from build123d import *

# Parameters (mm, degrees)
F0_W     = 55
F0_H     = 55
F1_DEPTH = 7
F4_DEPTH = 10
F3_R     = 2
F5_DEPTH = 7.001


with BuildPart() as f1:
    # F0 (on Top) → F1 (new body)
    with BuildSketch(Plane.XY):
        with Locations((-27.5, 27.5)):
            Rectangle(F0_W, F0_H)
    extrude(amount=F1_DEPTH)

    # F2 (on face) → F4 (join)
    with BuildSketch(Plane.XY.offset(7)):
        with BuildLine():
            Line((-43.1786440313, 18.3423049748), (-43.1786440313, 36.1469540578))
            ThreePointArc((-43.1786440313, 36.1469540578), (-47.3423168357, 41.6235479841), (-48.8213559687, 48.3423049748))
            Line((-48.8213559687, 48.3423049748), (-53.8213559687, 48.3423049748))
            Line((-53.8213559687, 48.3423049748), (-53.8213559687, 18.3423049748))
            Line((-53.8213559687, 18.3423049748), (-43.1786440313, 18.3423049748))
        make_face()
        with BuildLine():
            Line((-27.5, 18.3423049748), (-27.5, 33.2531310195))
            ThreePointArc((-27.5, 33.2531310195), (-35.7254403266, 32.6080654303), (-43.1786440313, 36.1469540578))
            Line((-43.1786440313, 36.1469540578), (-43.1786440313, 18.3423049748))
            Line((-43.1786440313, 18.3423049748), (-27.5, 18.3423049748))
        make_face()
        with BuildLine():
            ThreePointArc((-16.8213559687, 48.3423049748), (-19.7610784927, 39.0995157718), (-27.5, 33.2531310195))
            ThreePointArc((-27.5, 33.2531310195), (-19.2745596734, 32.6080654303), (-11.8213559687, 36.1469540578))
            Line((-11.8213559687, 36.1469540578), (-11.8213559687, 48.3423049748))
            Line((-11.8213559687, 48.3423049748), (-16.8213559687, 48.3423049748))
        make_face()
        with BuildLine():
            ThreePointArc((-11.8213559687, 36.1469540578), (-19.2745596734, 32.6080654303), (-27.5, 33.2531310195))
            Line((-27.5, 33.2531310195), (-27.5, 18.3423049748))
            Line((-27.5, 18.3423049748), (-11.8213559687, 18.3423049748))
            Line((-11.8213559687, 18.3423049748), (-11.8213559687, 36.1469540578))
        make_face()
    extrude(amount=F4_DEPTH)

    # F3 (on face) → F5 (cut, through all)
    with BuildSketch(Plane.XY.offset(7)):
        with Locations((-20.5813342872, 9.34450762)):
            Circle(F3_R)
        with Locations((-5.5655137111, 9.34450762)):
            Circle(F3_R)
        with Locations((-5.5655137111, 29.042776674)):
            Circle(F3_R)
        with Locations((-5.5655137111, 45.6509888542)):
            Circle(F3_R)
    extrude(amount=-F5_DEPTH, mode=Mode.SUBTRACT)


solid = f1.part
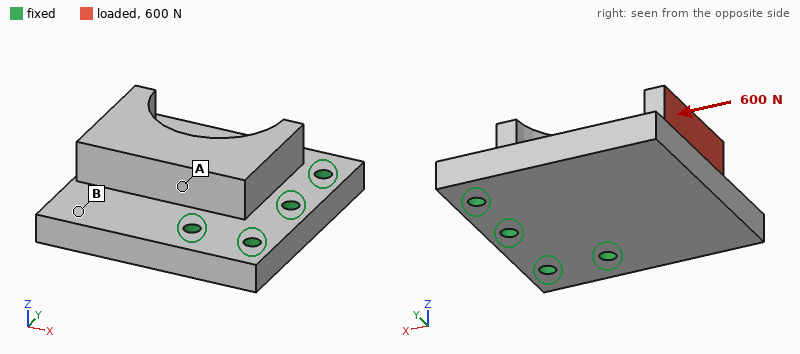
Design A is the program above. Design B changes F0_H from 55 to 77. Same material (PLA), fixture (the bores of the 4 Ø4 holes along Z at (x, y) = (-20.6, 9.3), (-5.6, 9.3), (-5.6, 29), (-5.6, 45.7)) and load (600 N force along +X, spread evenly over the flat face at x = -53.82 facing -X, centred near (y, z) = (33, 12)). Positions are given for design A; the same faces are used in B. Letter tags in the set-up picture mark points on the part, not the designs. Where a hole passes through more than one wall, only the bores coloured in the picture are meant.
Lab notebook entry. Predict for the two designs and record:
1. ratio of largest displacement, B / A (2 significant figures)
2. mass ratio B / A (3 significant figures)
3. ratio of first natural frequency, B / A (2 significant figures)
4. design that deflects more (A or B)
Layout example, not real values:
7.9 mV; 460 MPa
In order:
0.92; 1.29; 0.92; A
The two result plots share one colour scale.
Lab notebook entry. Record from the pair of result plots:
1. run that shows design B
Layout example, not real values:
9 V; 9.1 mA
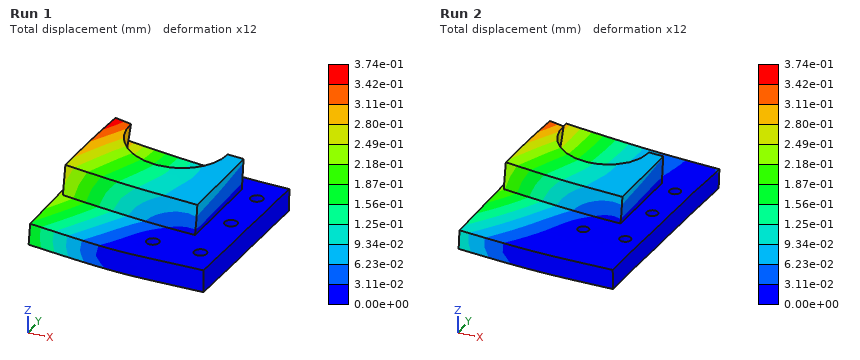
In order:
Run 2
